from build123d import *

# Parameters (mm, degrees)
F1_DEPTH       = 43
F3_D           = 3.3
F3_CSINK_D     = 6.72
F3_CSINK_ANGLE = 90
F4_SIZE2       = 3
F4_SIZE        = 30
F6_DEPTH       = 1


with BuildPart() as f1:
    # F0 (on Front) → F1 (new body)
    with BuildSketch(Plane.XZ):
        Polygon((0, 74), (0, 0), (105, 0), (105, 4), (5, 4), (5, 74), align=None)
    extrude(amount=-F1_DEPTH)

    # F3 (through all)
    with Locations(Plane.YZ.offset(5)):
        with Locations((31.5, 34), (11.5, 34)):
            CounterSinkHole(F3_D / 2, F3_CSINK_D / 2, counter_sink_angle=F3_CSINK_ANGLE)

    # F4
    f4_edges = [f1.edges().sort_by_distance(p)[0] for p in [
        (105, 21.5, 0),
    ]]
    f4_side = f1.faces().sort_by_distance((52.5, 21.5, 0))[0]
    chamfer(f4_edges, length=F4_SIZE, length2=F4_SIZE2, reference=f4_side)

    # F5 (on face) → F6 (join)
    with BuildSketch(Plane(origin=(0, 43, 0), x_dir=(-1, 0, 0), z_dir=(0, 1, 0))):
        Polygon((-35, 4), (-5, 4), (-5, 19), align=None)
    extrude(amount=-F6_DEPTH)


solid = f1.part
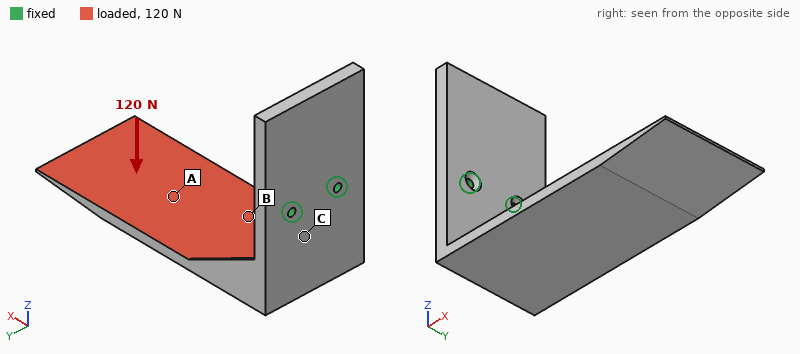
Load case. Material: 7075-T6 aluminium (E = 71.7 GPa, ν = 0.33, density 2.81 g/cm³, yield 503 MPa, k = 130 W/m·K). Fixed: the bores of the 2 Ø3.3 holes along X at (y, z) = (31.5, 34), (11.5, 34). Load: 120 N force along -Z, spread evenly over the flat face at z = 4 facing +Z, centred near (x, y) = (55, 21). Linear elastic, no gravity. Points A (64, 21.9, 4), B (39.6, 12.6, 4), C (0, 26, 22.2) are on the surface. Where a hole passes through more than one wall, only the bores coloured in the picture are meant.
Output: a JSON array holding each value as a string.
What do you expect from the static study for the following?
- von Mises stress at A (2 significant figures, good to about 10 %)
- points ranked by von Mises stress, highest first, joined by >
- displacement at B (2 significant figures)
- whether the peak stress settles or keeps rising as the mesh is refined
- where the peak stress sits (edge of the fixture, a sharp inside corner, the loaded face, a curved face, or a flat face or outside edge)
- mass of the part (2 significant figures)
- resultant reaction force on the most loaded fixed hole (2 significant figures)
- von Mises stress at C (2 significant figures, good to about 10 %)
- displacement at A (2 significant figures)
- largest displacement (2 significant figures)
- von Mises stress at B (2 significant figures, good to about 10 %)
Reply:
["10 MPa", "C > B > A", "0.38 mm", "keeps rising", "edge of the fixture", "88 g", "78 N", "32 MPa", "0.71 mm", "1.4 mm", "20 MPa"]
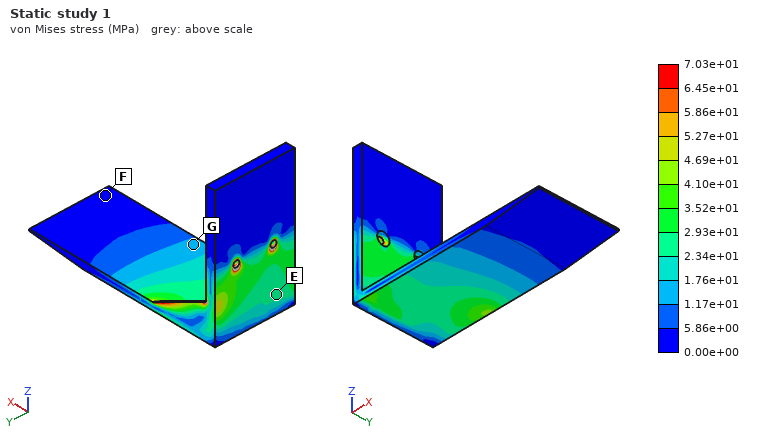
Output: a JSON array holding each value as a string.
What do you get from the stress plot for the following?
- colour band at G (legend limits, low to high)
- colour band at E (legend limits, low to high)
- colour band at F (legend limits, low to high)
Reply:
["1.17e+01 to 1.76e+01 MPa", "2.34e+01 to 2.93e+01 MPa", "0.00e+00 to 5.86e+00 MPa"]
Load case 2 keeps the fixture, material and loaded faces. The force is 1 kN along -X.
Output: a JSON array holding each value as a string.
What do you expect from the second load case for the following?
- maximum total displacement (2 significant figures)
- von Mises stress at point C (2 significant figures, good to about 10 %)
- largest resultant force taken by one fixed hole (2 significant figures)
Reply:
["1.6 mm", "91 MPa", "510 N"]
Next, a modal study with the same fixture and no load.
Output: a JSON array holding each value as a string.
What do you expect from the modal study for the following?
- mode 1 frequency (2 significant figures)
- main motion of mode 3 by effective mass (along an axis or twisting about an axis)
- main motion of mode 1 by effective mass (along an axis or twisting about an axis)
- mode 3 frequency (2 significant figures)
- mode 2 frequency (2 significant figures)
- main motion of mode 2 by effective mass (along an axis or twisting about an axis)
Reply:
["320 Hz", "along X", "along Z", "1200 Hz", "630 Hz", "along Y"]
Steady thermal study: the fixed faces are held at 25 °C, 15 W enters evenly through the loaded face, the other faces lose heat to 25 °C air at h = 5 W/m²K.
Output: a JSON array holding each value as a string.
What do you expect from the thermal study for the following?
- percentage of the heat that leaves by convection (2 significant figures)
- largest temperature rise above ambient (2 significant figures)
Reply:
["8.0 %", "49 K"]
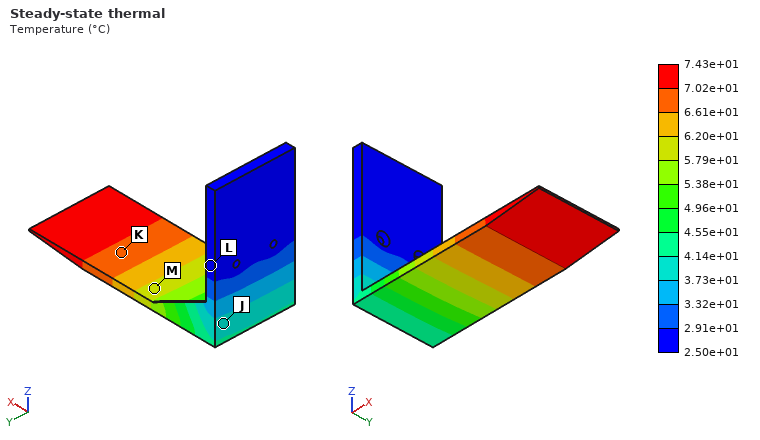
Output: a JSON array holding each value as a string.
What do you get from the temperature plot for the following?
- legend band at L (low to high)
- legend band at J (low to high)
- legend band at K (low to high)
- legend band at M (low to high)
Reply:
["2.50e+01 to 2.91e+01 °C", "3.73e+01 to 4.14e+01 °C", "6.61e+01 to 7.02e+01 °C", "5.79e+01 to 6.20e+01 °C"]
